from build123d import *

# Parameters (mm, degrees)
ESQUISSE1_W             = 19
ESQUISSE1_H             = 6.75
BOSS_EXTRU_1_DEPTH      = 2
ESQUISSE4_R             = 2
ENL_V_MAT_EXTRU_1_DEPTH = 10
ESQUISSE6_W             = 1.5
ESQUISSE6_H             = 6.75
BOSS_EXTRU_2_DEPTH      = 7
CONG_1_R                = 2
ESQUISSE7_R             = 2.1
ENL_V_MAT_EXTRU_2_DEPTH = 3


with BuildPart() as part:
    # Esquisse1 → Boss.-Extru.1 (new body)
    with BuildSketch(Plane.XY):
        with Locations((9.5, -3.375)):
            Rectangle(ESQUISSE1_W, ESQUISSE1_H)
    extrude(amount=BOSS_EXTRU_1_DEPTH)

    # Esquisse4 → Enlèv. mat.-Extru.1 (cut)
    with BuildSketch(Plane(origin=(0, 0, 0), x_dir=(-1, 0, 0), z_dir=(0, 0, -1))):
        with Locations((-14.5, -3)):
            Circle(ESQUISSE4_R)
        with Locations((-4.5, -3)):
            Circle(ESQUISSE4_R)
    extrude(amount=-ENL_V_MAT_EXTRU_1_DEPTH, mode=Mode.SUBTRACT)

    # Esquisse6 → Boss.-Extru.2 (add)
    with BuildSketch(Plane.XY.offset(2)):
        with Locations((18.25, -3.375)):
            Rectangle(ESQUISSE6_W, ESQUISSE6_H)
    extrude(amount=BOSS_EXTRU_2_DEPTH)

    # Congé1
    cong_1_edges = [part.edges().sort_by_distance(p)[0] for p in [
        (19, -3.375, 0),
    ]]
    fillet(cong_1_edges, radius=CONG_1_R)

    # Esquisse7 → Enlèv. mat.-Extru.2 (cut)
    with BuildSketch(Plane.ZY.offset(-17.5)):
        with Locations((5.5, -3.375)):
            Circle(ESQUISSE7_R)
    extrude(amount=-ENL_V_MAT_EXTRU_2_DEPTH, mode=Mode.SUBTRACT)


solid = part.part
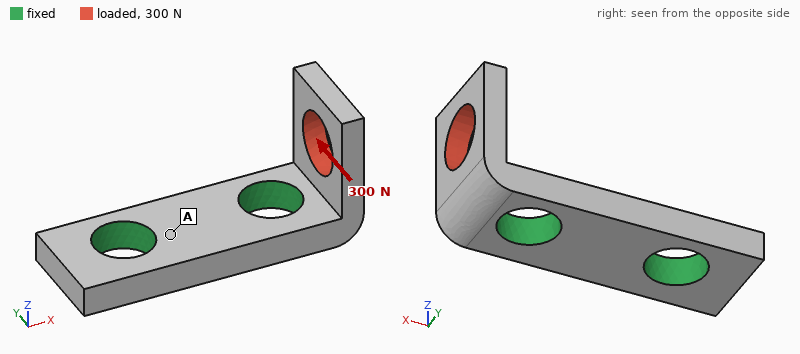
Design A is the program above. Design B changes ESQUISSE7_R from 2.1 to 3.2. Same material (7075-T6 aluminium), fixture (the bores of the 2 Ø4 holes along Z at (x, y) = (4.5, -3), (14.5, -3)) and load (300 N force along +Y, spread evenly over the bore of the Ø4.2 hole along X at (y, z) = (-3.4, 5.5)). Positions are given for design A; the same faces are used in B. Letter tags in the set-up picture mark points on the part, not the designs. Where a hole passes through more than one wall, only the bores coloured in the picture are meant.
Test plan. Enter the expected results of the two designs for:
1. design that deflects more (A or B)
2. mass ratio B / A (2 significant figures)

B
0.89
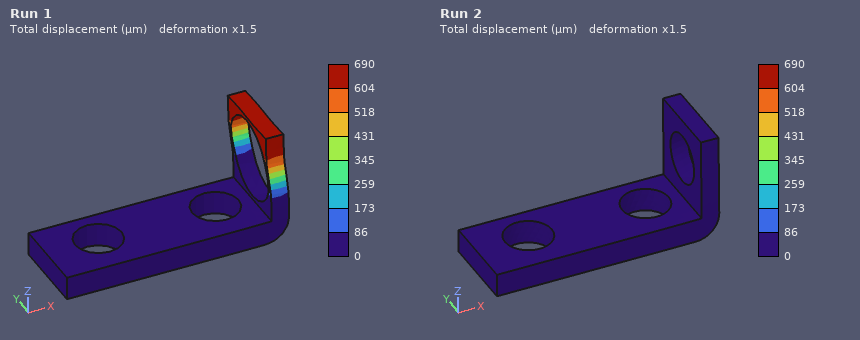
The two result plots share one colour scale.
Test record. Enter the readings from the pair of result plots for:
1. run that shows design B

Run 1
